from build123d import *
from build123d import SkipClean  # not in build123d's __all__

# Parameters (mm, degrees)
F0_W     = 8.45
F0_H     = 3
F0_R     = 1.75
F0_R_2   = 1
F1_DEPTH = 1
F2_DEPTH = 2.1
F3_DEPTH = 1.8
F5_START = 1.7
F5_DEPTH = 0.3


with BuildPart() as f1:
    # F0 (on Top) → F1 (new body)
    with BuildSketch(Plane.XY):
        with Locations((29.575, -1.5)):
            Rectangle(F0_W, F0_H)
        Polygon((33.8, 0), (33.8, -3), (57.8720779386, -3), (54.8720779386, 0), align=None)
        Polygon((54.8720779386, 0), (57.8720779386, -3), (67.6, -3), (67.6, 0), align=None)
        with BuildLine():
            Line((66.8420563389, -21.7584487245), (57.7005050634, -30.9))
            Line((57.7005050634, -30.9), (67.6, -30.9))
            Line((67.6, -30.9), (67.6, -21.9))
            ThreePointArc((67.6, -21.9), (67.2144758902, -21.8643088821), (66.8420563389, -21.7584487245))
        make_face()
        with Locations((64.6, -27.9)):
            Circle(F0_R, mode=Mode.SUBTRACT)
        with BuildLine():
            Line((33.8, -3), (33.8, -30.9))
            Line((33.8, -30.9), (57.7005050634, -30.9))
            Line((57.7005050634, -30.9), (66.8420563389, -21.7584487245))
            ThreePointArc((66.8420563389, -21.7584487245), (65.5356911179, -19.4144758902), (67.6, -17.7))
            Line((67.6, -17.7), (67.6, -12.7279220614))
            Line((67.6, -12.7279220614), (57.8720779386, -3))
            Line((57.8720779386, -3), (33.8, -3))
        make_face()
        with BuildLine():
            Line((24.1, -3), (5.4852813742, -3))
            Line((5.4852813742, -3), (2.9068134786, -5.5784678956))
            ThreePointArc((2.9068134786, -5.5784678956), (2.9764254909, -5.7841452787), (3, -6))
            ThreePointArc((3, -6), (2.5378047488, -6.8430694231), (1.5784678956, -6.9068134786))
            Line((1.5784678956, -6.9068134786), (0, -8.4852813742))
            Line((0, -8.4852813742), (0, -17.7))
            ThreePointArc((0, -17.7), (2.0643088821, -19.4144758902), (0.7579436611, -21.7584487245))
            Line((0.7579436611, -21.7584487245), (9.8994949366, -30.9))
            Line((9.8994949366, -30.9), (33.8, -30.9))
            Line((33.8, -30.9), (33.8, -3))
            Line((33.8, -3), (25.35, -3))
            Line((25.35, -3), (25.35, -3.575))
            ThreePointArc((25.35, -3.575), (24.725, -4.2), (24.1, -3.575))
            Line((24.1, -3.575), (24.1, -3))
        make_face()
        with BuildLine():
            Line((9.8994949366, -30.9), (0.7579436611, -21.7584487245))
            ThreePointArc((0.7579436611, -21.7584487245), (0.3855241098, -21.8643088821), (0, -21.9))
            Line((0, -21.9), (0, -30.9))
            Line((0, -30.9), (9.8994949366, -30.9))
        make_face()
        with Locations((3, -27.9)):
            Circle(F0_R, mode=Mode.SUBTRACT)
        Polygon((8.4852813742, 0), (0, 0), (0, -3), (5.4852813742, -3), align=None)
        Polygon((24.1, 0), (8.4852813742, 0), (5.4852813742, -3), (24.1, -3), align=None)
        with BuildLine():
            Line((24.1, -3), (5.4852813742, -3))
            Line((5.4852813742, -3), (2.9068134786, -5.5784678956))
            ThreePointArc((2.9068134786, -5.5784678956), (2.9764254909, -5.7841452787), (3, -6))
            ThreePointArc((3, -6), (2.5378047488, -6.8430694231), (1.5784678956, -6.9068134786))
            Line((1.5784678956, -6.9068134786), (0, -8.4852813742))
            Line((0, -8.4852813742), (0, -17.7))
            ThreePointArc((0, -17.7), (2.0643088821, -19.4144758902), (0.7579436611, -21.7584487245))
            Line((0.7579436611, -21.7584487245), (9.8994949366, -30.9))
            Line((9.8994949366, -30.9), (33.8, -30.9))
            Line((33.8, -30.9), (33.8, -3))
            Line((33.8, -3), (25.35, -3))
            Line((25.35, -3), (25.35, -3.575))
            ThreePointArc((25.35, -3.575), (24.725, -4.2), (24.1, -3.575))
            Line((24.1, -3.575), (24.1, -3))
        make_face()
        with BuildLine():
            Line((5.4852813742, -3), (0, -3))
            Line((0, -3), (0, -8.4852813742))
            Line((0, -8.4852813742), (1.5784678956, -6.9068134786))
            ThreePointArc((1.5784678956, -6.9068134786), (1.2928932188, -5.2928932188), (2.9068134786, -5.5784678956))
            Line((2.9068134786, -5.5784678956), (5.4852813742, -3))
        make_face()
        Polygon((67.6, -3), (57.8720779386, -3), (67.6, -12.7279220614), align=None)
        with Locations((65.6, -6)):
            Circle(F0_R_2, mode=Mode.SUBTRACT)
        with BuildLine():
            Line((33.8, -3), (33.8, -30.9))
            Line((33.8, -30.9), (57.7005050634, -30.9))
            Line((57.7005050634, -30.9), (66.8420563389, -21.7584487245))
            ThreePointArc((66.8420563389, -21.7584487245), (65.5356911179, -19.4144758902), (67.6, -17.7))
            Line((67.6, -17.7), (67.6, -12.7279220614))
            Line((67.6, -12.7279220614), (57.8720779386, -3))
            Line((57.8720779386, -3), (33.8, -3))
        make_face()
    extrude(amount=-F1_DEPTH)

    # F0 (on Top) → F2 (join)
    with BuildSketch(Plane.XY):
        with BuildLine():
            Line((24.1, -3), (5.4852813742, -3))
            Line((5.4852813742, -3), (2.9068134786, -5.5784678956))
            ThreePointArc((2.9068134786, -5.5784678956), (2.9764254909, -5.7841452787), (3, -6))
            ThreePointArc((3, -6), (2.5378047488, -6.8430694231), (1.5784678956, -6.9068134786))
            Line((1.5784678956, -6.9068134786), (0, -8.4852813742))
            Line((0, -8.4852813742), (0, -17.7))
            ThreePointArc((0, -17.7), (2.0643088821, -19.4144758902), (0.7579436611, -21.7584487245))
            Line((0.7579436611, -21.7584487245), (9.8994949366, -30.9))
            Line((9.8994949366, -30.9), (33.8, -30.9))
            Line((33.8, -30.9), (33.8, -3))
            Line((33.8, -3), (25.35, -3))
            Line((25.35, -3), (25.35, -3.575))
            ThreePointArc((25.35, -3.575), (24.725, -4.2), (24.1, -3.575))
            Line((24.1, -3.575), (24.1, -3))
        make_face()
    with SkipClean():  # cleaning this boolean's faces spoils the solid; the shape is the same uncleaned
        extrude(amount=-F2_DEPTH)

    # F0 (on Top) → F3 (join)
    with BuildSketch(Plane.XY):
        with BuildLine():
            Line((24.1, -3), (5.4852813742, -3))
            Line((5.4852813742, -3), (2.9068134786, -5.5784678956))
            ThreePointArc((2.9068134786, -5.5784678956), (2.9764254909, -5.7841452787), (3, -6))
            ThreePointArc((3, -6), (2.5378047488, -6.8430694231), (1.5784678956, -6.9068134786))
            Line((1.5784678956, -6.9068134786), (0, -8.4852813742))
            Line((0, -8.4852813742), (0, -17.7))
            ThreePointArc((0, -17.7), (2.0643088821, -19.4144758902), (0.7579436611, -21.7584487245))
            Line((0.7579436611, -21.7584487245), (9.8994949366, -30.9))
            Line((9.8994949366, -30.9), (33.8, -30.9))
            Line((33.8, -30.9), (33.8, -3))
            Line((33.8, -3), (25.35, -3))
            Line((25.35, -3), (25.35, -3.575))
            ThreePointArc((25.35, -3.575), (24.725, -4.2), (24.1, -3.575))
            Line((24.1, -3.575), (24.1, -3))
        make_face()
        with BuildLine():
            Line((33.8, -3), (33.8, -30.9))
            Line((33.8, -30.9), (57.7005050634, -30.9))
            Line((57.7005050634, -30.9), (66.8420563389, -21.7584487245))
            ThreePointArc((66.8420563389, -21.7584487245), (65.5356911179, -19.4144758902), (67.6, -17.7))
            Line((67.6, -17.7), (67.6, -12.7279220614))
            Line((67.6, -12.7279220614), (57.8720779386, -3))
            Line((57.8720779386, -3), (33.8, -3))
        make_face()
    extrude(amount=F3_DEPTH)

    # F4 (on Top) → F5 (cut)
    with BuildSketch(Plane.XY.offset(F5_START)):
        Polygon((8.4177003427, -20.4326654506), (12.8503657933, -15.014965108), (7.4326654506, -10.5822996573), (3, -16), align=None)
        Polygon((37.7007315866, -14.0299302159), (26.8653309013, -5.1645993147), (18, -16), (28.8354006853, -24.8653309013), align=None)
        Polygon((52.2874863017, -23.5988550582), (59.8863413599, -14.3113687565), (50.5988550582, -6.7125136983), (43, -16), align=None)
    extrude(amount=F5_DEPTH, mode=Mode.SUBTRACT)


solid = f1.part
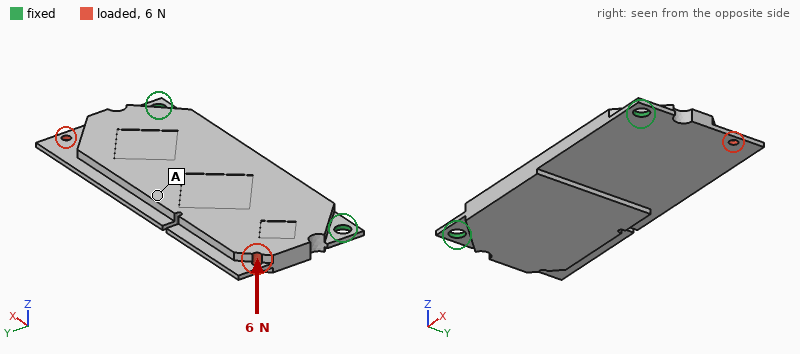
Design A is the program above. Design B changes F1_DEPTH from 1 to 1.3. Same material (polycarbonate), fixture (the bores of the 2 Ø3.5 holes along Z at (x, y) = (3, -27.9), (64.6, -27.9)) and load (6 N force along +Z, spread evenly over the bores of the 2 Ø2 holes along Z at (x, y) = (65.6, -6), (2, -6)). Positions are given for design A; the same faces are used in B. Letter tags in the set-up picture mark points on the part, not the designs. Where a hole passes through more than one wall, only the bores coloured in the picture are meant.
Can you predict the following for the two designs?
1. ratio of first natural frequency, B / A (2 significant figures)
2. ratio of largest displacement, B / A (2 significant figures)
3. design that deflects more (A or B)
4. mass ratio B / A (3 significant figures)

1.2
0.62
A
1.06
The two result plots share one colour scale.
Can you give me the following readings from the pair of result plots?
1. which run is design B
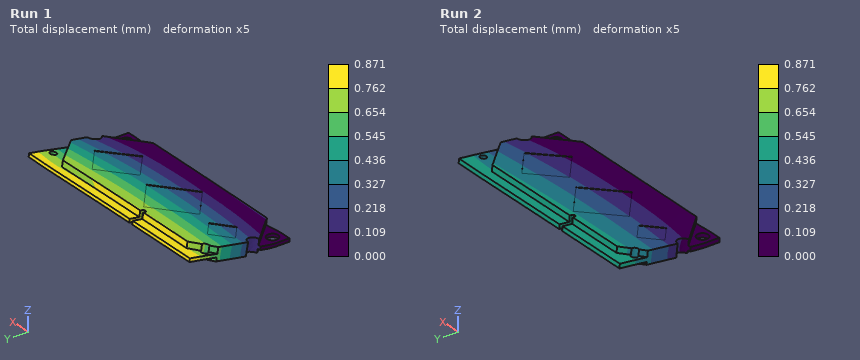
Run 2
